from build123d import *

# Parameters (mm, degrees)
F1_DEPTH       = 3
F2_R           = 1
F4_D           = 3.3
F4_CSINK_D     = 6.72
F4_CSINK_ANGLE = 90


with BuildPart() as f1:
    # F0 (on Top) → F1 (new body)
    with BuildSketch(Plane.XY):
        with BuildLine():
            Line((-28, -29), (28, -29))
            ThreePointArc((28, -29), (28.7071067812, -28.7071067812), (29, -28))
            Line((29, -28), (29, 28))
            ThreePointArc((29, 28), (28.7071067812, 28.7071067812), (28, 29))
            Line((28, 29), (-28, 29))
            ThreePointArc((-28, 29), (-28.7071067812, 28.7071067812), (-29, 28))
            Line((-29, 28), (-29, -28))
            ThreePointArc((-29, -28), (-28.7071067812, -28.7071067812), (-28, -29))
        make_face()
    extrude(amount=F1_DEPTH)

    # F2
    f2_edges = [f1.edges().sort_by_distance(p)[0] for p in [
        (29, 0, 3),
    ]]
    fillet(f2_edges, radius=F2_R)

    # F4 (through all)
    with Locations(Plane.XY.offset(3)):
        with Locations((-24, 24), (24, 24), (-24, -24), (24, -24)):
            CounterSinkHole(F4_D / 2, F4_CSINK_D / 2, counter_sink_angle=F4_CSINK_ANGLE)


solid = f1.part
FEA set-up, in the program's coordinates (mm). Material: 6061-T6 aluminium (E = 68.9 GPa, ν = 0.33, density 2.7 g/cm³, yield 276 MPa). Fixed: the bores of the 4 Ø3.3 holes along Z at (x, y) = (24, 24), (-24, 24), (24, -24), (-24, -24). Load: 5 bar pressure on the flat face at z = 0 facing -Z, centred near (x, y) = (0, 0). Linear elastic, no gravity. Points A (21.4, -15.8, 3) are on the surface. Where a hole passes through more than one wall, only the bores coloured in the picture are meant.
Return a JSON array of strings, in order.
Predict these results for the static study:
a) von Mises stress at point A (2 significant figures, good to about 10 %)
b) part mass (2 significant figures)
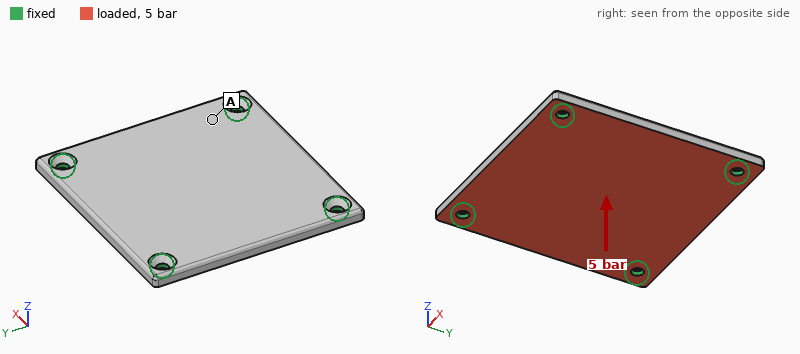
["31 MPa", "27 g"]
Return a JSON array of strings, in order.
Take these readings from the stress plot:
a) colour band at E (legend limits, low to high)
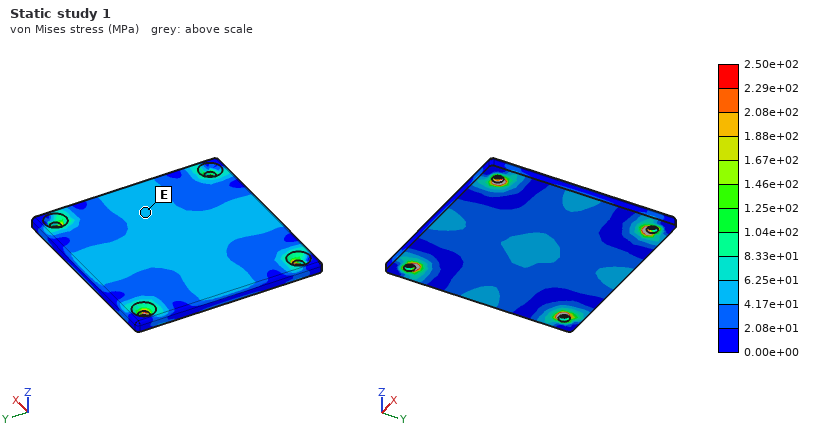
["4.17e+01 to 6.25e+01 MPa"]
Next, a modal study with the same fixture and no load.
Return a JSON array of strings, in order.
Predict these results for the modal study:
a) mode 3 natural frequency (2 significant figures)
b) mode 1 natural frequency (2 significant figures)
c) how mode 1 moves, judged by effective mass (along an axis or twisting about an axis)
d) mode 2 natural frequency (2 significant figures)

["6500 Hz", "3900 Hz", "along Z", "6500 Hz"]
